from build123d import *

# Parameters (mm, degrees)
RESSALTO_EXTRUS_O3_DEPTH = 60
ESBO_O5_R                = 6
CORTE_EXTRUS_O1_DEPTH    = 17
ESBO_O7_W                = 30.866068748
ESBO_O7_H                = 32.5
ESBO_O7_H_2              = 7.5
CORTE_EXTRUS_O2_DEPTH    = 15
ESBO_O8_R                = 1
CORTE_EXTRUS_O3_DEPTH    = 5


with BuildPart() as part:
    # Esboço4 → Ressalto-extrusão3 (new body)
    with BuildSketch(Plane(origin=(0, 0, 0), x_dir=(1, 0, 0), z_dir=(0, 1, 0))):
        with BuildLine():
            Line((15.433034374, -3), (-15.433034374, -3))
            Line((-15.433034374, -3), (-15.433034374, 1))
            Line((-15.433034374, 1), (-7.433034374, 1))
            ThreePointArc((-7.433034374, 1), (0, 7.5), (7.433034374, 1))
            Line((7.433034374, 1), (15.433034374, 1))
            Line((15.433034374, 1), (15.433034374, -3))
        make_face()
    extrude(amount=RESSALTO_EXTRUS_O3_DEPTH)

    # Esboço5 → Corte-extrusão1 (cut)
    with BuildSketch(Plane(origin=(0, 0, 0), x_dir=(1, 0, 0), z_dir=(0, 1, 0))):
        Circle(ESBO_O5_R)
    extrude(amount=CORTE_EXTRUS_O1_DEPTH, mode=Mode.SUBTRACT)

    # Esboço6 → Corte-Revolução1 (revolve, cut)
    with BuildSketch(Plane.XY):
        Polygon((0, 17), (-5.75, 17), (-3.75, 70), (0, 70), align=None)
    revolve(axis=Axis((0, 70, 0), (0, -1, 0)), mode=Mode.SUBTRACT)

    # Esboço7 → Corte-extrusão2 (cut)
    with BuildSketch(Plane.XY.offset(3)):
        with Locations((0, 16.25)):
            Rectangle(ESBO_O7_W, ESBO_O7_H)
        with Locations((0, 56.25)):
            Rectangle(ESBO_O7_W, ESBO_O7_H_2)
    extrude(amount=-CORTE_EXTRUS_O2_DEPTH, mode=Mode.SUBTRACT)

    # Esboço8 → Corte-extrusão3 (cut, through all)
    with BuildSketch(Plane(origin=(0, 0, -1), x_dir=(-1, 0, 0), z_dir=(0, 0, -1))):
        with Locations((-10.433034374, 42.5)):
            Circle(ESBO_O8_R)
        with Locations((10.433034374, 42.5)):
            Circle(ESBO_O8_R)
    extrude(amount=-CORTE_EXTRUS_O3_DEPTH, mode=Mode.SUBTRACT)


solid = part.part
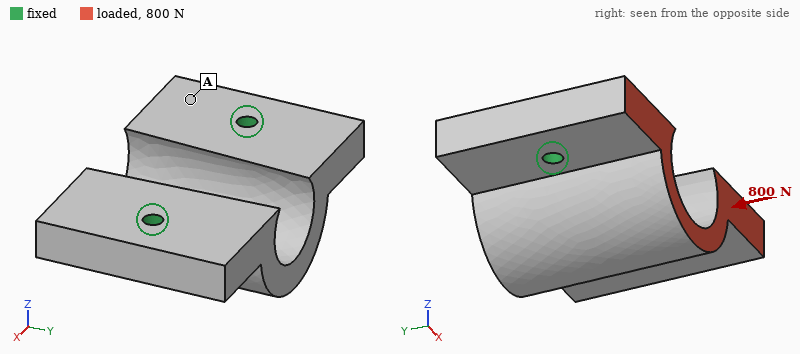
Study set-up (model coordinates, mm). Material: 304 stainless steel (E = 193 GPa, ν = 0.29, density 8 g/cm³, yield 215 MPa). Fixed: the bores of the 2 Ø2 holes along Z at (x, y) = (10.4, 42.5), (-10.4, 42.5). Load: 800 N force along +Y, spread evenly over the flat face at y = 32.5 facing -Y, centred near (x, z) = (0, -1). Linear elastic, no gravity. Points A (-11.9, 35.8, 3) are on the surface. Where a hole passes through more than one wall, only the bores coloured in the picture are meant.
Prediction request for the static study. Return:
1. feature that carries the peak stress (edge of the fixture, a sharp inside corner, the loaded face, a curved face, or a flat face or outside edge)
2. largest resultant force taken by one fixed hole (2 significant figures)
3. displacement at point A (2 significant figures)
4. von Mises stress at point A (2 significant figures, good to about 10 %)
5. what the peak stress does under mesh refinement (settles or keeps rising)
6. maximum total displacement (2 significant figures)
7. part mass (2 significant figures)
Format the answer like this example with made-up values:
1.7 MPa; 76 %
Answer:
edge of the fixture; 400 N; 1.2 µm; 8.5 MPa; keeps rising; 4.5 µm; 21 g
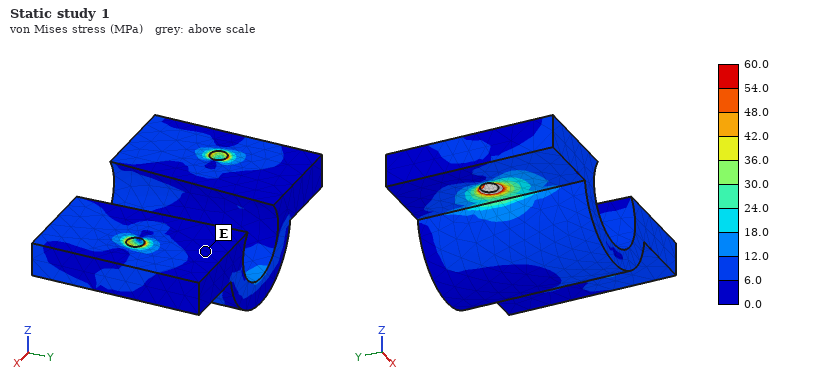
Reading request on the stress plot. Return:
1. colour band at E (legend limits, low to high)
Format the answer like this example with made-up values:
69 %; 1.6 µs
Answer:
0.0 to 6.0 MPa
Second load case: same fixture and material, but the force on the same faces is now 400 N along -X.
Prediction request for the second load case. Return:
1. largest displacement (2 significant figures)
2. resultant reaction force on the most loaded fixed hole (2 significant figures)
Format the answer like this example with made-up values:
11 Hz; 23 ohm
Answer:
3.3 µm; 240 N
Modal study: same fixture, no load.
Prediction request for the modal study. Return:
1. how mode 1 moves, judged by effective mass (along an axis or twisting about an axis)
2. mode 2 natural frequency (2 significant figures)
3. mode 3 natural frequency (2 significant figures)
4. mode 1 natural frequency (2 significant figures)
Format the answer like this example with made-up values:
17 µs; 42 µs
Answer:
along Y; 22 kHz; 24 kHz; 14 kHz
